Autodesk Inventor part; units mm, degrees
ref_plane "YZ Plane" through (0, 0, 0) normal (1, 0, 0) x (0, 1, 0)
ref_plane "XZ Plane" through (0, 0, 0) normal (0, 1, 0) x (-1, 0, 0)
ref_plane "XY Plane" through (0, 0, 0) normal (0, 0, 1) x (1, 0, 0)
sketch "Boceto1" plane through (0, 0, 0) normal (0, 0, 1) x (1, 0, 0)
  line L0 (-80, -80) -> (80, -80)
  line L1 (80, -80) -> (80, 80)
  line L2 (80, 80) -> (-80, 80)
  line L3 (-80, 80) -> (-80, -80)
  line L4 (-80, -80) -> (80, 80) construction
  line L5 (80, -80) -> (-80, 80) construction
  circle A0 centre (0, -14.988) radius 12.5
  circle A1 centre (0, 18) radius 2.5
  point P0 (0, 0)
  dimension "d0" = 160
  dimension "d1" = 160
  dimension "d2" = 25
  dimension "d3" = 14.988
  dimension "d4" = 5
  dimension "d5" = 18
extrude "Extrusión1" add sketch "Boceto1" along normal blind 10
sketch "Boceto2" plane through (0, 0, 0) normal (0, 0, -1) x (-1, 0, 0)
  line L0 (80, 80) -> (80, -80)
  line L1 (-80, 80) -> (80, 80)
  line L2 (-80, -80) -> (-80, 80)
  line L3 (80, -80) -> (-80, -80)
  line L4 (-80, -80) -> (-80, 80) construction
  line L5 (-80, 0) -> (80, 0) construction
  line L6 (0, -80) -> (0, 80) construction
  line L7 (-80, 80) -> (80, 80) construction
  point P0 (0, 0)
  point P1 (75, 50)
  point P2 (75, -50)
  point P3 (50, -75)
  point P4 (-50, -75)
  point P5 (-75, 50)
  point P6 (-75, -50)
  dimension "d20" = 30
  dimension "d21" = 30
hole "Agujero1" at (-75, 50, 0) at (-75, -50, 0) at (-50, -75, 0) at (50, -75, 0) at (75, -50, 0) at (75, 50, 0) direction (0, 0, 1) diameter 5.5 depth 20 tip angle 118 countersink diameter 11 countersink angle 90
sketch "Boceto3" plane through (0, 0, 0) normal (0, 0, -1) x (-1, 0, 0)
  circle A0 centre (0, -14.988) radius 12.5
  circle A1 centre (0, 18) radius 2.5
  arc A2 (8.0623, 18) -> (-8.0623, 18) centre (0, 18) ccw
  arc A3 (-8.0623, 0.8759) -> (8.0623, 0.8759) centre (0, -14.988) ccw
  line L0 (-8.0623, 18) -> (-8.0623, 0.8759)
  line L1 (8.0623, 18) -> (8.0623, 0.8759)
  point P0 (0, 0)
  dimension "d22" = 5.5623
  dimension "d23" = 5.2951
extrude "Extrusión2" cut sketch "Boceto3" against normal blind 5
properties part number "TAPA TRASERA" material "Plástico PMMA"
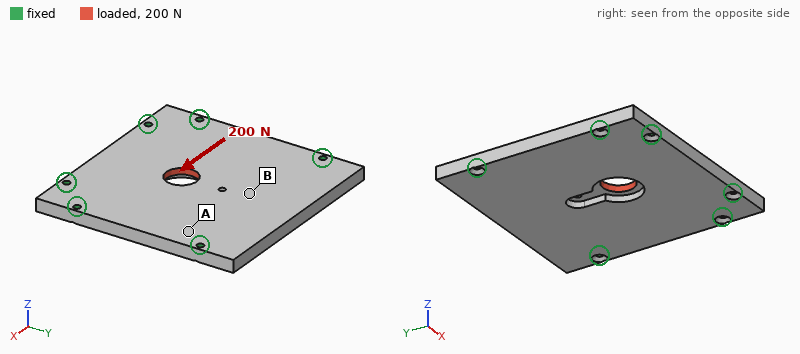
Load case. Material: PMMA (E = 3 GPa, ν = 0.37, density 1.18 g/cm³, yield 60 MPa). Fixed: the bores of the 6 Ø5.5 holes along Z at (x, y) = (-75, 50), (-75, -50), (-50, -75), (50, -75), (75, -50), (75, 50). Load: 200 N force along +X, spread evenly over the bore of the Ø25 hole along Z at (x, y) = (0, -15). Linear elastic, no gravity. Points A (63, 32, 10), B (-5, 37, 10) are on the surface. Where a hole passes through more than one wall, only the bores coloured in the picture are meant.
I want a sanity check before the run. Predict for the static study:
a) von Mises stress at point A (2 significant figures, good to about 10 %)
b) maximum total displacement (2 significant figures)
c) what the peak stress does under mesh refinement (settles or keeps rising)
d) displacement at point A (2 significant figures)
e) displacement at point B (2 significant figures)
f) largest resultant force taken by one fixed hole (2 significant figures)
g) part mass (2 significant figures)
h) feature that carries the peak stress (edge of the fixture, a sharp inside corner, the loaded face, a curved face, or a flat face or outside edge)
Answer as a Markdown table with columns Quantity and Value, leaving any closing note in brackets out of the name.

| Quantity | Value |
|---|---|
| von Mises stress at point A | 0.15 MPa |
| maximum total displacement | 7.3 µm |
| what the peak stress does under mesh refinement | keeps rising |
| displacement at point A | 2.2 µm |
| displacement at point B | 2.4 µm |
| largest resultant force taken by one fixed hole | 41 N |
| part mass | 290 g |
| feature that carries the peak stress | edge of the fixture |
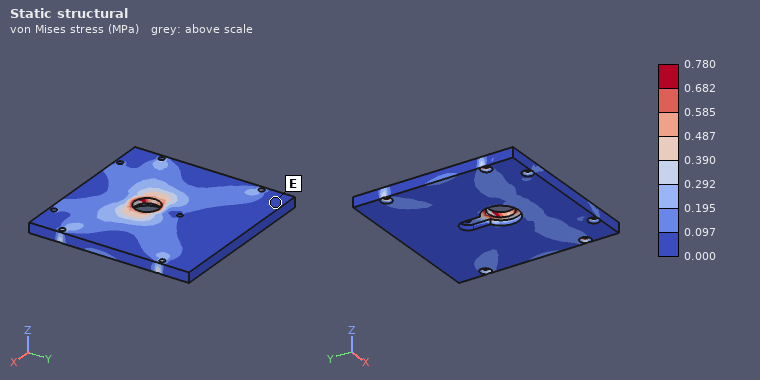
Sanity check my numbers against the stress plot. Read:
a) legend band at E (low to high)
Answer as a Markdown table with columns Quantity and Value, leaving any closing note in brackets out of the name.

| Quantity | Value |
|---|---|
| legend band at E | 0.000 to 0.097 MPa |
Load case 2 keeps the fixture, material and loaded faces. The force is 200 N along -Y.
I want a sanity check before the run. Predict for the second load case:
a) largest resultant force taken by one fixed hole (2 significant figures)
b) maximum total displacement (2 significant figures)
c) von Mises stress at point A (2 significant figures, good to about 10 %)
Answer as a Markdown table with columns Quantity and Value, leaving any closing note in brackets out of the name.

| Quantity | Value |
|---|---|
| largest resultant force taken by one fixed hole | 49 N |
| maximum total displacement | 8.4 µm |
| von Mises stress at point A | 0.14 MPa |
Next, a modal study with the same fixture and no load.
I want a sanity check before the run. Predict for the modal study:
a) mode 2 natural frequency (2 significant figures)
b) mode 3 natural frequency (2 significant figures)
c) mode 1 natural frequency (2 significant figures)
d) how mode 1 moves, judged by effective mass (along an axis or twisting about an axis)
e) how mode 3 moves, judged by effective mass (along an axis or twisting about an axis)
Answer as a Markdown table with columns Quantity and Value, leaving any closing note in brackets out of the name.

| Quantity | Value |
|---|---|
| mode 2 natural frequency | 780 Hz |
| mode 3 natural frequency | 1200 Hz |
| mode 1 natural frequency | 520 Hz |
| how mode 1 moves, judged by effective mass | along Z |
| how mode 3 moves, judged by effective mass | twisting about Y |
